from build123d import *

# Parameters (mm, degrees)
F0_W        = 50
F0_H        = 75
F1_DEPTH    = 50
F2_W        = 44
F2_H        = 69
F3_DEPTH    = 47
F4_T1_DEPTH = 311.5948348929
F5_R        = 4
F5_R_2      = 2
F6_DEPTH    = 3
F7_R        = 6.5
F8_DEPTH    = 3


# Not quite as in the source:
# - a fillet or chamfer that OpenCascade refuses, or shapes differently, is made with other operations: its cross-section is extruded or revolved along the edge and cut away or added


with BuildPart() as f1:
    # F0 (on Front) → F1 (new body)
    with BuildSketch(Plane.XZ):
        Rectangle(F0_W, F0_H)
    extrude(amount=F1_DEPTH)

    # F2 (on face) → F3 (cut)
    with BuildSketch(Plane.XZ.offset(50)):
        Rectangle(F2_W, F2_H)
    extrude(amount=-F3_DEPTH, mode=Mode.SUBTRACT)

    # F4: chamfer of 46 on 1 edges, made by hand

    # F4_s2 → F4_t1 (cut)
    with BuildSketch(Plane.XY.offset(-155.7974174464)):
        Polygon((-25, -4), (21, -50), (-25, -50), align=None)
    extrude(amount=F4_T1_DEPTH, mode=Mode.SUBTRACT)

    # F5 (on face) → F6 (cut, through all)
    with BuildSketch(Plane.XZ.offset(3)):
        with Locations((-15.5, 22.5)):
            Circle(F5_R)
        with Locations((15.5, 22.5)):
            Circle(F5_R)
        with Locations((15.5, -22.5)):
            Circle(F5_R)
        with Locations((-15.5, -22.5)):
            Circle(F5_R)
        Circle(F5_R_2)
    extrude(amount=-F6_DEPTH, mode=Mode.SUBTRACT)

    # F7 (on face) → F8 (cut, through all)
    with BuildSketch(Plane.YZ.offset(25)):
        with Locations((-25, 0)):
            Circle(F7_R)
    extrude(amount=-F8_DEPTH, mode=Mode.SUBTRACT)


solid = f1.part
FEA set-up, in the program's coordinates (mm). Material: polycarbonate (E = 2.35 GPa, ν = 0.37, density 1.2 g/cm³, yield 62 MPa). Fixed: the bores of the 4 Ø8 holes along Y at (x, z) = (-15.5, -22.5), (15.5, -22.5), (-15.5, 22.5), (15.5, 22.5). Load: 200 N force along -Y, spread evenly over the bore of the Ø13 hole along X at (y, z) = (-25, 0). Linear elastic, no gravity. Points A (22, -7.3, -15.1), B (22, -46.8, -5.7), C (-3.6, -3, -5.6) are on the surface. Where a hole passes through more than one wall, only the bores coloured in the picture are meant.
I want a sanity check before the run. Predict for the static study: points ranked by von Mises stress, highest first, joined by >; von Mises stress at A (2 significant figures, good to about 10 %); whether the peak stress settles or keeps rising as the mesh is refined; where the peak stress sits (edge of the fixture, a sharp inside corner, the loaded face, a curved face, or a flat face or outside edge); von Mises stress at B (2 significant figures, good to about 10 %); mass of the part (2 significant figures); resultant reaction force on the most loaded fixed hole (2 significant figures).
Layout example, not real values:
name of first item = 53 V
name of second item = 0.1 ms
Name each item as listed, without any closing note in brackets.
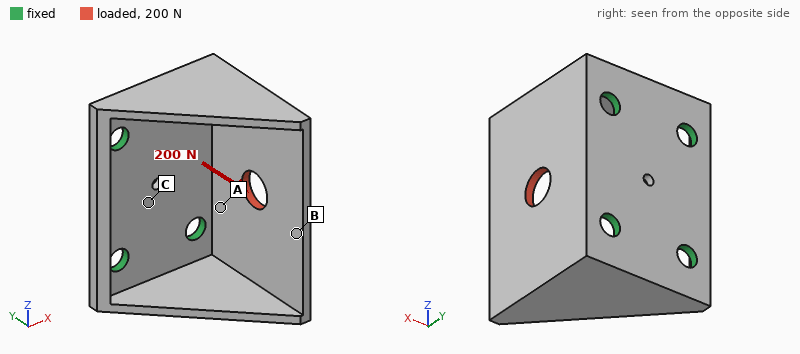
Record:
points ranked by von Mises stress, highest first, joined by > = A > B > C
von Mises stress at A = 2.7 MPa
whether the peak stress settles or keeps rising as the mesh is refined = keeps rising
where the peak stress sits = edge of the fixture
von Mises stress at B = 1.5 MPa
mass of the part = 34 g
resultant reaction force on the most loaded fixed hole = 110 N
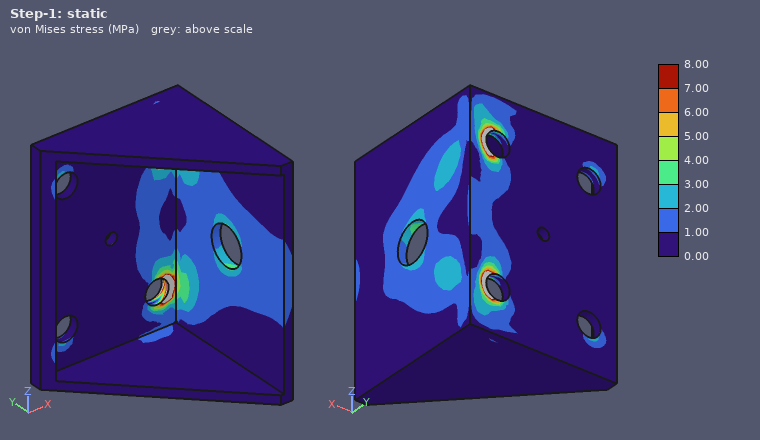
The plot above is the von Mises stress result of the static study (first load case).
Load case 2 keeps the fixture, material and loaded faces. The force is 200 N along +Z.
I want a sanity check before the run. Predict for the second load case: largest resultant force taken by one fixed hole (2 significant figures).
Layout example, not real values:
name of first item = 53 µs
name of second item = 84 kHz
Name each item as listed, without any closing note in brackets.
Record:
largest resultant force taken by one fixed hole = 140 N
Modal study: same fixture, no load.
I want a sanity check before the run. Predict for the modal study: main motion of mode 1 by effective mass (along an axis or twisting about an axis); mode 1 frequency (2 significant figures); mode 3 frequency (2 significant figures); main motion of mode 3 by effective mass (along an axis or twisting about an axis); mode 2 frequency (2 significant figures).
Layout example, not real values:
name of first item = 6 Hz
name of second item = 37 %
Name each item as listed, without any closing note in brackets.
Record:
main motion of mode 1 by effective mass = along X
mode 1 frequency = 620 Hz
mode 3 frequency = 1300 Hz
main motion of mode 3 by effective mass = along Z
mode 2 frequency = 1200 Hz
